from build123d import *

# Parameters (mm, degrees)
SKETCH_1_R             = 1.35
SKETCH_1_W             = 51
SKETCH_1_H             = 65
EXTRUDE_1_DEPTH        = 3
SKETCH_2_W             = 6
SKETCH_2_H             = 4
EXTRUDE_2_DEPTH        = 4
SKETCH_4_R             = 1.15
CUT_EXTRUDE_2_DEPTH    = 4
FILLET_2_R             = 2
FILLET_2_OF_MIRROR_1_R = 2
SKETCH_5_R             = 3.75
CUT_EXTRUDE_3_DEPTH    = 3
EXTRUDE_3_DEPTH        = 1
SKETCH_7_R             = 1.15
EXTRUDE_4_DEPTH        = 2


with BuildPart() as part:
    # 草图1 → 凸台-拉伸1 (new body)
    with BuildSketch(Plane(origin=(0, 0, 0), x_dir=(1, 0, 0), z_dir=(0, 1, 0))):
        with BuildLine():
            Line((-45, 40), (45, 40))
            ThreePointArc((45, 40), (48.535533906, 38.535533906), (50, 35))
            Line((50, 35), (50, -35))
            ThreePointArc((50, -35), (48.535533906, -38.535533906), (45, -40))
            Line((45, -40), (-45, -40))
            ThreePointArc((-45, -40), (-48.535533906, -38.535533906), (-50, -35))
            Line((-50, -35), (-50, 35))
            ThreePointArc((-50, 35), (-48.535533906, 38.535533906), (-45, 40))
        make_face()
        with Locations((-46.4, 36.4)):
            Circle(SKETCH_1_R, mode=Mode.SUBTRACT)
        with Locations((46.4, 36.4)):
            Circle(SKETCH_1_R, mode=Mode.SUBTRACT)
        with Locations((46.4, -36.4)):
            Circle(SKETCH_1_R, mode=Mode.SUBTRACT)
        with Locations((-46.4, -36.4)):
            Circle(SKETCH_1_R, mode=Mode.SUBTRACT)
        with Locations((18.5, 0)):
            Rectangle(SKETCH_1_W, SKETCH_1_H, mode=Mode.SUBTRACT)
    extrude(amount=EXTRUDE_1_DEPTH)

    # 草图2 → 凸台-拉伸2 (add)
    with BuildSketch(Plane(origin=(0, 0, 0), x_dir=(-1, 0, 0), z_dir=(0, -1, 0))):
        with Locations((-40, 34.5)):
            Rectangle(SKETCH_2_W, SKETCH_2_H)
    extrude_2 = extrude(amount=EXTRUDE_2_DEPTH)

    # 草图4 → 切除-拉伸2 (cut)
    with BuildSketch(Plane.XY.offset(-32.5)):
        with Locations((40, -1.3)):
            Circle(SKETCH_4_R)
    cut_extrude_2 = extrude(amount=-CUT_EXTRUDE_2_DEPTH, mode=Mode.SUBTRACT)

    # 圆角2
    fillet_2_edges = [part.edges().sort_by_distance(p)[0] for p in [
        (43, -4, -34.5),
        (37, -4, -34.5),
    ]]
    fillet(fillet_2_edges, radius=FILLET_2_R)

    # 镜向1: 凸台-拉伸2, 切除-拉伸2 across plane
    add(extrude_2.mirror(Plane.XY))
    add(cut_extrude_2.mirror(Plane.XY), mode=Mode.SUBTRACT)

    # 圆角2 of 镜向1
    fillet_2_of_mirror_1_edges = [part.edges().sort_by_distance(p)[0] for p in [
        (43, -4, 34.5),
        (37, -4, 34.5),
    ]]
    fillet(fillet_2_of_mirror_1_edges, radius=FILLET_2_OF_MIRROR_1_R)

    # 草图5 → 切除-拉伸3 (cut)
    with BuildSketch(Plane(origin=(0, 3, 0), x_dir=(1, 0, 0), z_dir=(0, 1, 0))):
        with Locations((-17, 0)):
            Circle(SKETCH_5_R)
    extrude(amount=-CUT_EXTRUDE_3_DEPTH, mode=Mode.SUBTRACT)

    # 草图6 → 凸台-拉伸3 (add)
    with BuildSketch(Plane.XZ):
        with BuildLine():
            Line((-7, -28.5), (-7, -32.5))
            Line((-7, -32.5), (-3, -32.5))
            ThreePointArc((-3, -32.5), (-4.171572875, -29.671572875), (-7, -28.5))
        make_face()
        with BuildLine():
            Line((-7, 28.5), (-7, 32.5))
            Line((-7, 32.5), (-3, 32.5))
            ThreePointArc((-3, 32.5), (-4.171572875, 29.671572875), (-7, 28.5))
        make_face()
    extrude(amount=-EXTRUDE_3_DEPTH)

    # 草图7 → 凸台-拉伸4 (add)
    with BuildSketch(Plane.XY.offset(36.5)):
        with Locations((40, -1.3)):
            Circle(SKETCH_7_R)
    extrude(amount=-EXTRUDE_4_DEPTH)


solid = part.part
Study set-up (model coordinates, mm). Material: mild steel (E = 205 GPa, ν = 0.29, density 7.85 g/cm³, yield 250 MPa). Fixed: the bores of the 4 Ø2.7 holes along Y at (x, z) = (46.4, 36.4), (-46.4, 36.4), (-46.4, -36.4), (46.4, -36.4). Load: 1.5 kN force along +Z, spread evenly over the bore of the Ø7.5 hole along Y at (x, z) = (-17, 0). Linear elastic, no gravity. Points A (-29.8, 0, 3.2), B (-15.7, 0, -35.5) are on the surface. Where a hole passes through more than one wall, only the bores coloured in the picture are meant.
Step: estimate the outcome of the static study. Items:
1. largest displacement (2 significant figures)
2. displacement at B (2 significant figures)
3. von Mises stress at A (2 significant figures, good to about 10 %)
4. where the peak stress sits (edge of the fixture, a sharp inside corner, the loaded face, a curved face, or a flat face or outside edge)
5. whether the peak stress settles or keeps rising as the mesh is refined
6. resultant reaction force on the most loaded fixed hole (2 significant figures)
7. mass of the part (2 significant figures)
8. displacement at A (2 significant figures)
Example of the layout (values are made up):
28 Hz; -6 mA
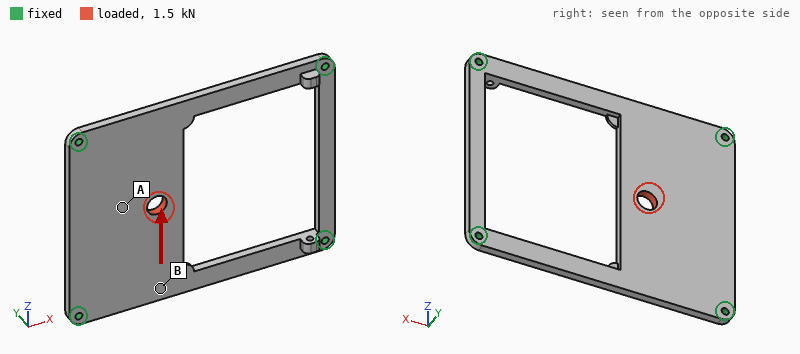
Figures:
5.6 µm; 4.1 µm; 14 MPa; edge of the fixture; keeps rising; 910 N; 110 g; 3.1 µm
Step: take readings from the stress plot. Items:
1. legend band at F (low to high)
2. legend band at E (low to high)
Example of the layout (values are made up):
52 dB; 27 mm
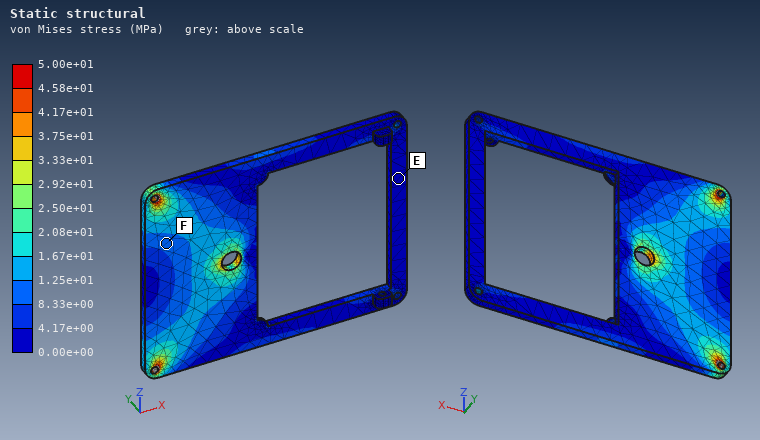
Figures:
8.33e+00 to 1.25e+01 MPa; 0.00e+00 to 4.17e+00 MPa
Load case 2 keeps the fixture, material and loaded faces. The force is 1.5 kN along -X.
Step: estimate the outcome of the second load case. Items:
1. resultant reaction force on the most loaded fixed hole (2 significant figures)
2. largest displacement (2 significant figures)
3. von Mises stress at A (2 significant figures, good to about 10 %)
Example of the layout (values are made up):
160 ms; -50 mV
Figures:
800 N; 6.5 µm; 11 MPa
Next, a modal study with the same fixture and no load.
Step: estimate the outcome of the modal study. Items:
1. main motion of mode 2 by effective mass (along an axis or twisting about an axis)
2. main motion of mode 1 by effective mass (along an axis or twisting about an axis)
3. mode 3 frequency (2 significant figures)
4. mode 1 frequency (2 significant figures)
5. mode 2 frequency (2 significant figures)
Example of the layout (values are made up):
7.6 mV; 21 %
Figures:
twisting about X; along Y; 2600 Hz; 1300 Hz; 2100 Hz
